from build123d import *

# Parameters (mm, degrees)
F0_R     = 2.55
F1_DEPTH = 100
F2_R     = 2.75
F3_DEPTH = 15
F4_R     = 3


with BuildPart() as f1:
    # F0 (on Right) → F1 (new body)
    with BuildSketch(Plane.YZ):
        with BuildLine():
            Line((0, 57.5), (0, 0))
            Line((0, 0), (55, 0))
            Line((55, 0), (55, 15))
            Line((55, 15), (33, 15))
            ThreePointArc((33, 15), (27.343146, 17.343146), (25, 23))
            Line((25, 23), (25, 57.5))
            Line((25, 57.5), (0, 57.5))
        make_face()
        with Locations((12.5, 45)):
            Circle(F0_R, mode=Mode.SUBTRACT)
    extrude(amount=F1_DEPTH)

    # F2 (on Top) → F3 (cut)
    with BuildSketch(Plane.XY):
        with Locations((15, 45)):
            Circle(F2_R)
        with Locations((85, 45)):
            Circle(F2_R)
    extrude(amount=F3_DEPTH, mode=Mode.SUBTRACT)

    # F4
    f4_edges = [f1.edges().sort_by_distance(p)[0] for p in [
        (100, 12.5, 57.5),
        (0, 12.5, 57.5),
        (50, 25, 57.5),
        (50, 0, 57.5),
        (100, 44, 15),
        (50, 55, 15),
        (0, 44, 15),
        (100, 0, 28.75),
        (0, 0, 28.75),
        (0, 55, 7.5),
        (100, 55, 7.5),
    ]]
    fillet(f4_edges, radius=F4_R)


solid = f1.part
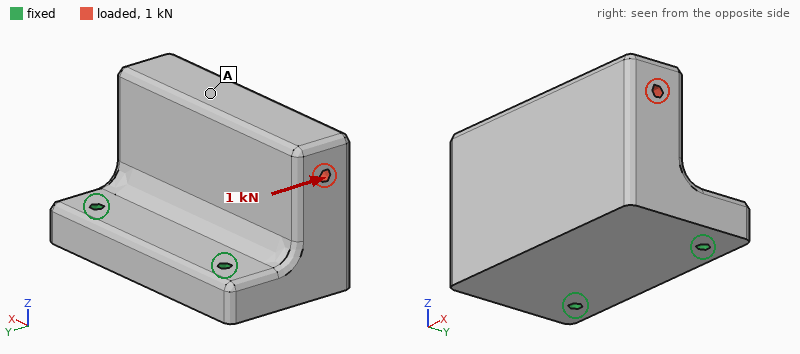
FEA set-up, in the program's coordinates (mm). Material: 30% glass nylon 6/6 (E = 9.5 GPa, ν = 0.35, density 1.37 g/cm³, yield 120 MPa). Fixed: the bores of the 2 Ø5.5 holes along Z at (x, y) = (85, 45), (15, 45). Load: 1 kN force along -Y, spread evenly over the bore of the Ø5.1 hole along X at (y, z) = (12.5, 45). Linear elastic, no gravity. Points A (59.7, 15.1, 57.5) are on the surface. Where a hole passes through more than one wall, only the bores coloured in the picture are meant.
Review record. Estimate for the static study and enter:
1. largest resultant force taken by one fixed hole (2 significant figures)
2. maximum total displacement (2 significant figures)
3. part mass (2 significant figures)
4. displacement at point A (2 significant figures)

520 N
0.30 mm
260 g
0.27 mm
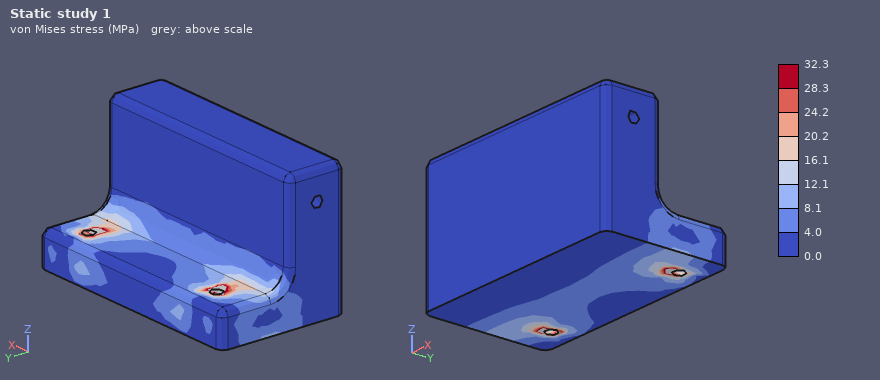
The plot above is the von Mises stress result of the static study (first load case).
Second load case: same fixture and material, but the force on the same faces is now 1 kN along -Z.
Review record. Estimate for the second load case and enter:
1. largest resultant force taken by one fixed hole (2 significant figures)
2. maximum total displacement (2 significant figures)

500 N
0.19 mm
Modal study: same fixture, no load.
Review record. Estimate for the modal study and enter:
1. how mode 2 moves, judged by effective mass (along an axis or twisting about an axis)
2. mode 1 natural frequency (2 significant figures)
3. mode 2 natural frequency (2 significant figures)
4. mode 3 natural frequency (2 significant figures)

along X
850 Hz
2100 Hz
3400 Hz
